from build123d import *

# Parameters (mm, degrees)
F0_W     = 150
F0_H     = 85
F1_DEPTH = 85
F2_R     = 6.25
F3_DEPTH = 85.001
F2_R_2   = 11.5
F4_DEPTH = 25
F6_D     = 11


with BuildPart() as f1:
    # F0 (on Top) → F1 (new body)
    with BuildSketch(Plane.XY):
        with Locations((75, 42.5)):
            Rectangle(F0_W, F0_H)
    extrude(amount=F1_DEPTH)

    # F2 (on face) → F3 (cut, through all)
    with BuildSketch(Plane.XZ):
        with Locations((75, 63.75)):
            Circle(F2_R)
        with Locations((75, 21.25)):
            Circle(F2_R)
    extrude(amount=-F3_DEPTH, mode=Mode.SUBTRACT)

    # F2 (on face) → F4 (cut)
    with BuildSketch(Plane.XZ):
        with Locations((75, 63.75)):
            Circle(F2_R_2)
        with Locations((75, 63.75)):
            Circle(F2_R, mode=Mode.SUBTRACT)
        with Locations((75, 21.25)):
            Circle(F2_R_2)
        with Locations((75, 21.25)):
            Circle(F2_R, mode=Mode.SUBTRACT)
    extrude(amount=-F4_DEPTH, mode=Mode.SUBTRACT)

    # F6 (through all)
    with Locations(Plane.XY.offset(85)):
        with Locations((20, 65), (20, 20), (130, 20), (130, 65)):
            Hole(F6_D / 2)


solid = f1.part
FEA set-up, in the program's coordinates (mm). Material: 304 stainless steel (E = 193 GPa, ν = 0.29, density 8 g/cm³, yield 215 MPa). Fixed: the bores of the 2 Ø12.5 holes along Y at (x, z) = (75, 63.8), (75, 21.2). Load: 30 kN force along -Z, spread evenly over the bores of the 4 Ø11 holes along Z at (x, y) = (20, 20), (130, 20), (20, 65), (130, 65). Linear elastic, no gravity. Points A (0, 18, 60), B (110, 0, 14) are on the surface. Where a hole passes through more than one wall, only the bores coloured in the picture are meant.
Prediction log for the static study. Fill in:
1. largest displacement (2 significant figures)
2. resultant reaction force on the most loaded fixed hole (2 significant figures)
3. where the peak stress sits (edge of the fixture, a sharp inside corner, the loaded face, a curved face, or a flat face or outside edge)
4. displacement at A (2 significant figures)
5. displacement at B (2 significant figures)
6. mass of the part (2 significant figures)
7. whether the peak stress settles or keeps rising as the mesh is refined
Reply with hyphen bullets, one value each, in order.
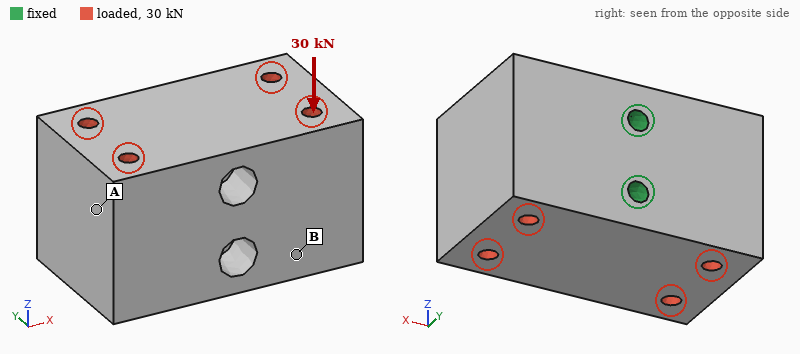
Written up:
- 4.2 µm
- 15 kN
- edge of the fixture
- 3.9 µm
- 2.4 µm
- 8.1 kg
- keeps rising
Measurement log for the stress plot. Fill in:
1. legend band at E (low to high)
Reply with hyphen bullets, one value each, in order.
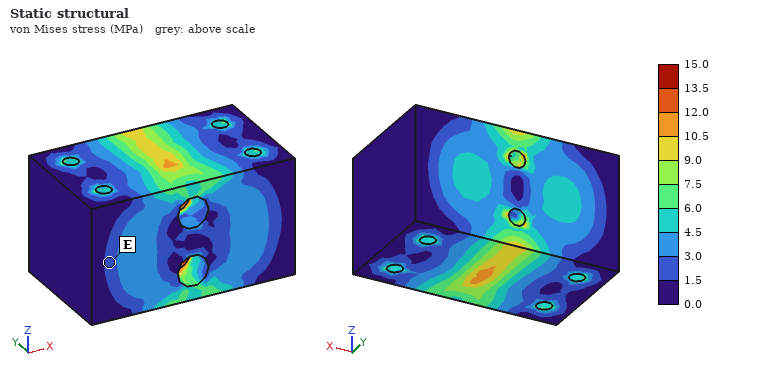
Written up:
- 1.5 to 3.0 MPa
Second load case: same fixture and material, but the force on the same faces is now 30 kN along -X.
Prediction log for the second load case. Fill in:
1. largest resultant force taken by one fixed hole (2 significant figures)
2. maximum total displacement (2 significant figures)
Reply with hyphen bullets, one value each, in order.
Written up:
- 15 kN
- 2.3 µm
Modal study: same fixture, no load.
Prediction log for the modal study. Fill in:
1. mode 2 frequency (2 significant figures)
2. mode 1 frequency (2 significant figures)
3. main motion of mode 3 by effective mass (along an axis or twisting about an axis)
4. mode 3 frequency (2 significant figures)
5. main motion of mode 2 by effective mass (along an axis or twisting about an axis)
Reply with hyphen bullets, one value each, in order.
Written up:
- 5300 Hz
- 4600 Hz
- along Z
- 6700 Hz
- twisting about Y
